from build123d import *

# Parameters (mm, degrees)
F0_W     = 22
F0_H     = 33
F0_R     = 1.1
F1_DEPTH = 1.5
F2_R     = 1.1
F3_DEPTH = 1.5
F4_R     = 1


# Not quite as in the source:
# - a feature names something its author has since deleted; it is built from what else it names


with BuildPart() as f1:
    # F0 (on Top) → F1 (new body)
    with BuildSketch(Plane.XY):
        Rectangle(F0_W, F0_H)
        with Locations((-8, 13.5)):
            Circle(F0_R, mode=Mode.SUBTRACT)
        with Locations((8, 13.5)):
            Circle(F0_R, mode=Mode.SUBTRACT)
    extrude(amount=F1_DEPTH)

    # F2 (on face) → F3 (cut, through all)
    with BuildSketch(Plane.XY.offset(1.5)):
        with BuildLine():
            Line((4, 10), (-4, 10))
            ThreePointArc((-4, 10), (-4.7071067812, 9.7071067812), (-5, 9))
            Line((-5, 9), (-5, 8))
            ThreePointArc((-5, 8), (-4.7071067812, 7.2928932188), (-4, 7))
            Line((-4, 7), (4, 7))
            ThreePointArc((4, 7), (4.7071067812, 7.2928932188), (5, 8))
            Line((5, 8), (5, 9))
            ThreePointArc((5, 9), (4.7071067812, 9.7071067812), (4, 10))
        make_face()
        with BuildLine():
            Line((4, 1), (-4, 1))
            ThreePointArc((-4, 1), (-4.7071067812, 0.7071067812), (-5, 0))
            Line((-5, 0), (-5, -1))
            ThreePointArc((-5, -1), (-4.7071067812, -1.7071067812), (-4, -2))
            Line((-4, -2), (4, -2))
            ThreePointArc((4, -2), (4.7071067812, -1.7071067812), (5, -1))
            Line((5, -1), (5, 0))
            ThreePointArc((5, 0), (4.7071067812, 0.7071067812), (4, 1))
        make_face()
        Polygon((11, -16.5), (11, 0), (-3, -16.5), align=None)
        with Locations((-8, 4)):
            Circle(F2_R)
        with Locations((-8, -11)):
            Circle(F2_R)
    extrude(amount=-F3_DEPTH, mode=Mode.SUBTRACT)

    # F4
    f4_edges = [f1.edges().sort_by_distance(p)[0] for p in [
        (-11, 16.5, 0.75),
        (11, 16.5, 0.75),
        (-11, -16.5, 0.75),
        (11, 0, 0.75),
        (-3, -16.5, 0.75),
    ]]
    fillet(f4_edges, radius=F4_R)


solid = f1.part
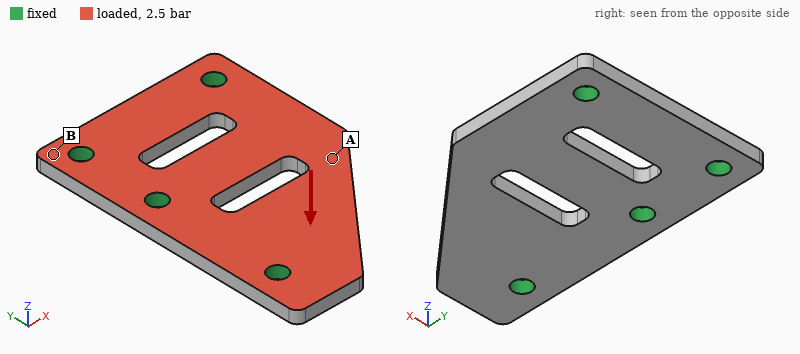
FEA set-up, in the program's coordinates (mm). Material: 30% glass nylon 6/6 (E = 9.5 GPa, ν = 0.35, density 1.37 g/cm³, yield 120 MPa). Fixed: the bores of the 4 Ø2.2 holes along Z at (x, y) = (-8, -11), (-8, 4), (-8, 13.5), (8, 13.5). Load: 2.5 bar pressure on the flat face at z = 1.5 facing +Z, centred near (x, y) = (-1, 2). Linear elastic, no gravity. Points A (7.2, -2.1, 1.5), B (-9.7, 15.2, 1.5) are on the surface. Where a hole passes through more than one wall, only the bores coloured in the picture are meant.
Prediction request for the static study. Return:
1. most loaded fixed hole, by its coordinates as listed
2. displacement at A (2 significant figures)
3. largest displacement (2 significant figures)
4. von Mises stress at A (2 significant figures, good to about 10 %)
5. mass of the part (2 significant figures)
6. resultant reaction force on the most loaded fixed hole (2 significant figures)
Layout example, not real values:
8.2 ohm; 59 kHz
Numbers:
(-8, -11); 0.27 mm; 0.30 mm; 21 MPa; 1.1 g; 44 N
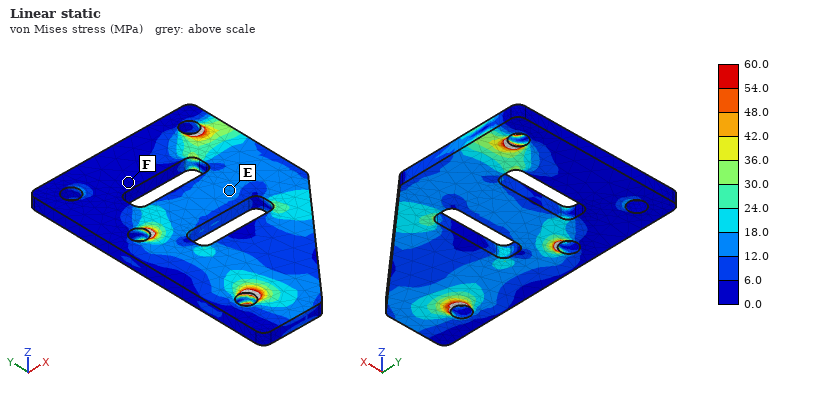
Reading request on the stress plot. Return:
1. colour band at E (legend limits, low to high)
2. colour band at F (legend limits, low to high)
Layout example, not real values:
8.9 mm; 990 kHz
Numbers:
12.0 to 18.0 MPa; 0.0 to 6.0 MPa
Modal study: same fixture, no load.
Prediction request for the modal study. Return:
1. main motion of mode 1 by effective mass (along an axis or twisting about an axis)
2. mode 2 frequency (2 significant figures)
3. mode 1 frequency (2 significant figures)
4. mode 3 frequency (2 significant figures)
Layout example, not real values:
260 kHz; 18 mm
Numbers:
along Z; 9900 Hz; 4300 Hz; 14 kHz
